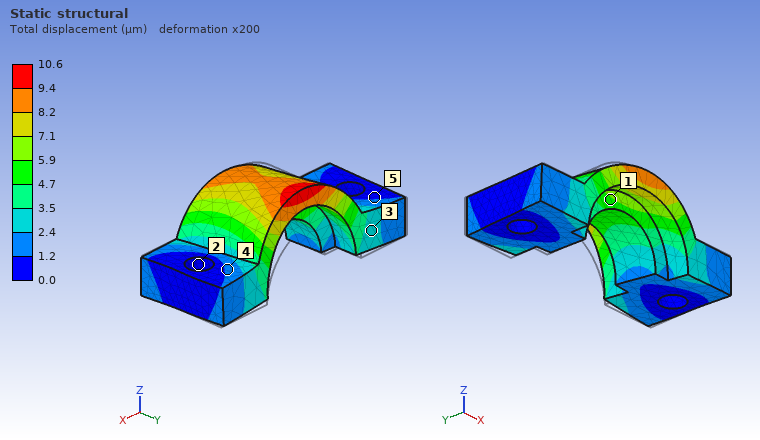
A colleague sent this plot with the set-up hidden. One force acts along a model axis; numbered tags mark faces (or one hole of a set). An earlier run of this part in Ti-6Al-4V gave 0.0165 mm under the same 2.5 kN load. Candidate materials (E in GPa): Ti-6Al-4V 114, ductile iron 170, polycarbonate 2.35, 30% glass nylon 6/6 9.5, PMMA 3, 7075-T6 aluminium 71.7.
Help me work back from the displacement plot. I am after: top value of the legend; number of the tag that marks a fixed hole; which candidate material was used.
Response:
10.6 µm
2
ductile iron
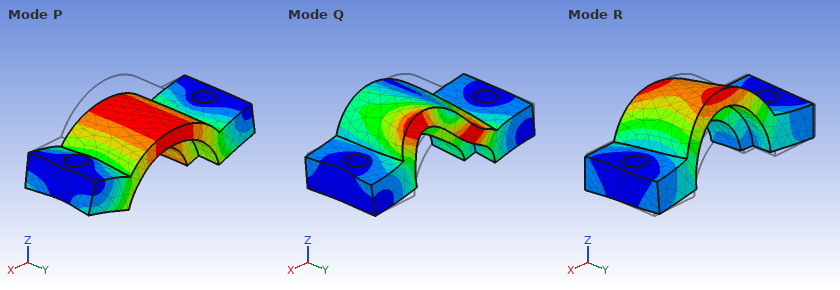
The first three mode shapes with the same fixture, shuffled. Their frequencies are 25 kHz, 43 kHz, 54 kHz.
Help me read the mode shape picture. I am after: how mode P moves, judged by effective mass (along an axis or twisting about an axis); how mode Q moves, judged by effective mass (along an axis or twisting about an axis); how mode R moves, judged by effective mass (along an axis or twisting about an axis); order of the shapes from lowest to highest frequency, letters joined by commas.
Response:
along Z
along X
along Y
R, P, Q
